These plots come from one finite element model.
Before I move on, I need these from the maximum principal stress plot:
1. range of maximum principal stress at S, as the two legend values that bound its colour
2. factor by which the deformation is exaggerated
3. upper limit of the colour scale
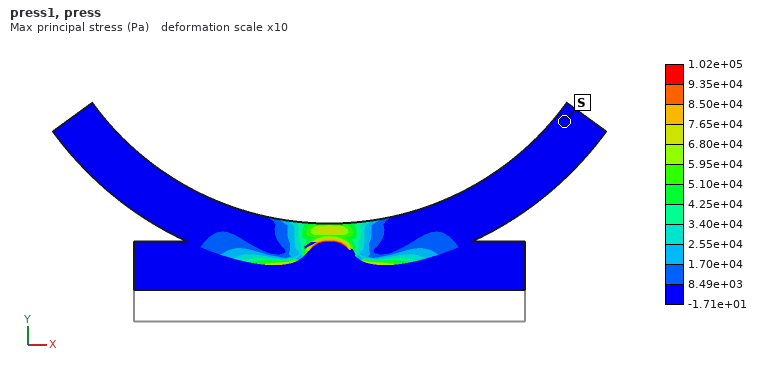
-1.71e+01 to 8.49e+03 Pa
10
1.02e+05 Pa
